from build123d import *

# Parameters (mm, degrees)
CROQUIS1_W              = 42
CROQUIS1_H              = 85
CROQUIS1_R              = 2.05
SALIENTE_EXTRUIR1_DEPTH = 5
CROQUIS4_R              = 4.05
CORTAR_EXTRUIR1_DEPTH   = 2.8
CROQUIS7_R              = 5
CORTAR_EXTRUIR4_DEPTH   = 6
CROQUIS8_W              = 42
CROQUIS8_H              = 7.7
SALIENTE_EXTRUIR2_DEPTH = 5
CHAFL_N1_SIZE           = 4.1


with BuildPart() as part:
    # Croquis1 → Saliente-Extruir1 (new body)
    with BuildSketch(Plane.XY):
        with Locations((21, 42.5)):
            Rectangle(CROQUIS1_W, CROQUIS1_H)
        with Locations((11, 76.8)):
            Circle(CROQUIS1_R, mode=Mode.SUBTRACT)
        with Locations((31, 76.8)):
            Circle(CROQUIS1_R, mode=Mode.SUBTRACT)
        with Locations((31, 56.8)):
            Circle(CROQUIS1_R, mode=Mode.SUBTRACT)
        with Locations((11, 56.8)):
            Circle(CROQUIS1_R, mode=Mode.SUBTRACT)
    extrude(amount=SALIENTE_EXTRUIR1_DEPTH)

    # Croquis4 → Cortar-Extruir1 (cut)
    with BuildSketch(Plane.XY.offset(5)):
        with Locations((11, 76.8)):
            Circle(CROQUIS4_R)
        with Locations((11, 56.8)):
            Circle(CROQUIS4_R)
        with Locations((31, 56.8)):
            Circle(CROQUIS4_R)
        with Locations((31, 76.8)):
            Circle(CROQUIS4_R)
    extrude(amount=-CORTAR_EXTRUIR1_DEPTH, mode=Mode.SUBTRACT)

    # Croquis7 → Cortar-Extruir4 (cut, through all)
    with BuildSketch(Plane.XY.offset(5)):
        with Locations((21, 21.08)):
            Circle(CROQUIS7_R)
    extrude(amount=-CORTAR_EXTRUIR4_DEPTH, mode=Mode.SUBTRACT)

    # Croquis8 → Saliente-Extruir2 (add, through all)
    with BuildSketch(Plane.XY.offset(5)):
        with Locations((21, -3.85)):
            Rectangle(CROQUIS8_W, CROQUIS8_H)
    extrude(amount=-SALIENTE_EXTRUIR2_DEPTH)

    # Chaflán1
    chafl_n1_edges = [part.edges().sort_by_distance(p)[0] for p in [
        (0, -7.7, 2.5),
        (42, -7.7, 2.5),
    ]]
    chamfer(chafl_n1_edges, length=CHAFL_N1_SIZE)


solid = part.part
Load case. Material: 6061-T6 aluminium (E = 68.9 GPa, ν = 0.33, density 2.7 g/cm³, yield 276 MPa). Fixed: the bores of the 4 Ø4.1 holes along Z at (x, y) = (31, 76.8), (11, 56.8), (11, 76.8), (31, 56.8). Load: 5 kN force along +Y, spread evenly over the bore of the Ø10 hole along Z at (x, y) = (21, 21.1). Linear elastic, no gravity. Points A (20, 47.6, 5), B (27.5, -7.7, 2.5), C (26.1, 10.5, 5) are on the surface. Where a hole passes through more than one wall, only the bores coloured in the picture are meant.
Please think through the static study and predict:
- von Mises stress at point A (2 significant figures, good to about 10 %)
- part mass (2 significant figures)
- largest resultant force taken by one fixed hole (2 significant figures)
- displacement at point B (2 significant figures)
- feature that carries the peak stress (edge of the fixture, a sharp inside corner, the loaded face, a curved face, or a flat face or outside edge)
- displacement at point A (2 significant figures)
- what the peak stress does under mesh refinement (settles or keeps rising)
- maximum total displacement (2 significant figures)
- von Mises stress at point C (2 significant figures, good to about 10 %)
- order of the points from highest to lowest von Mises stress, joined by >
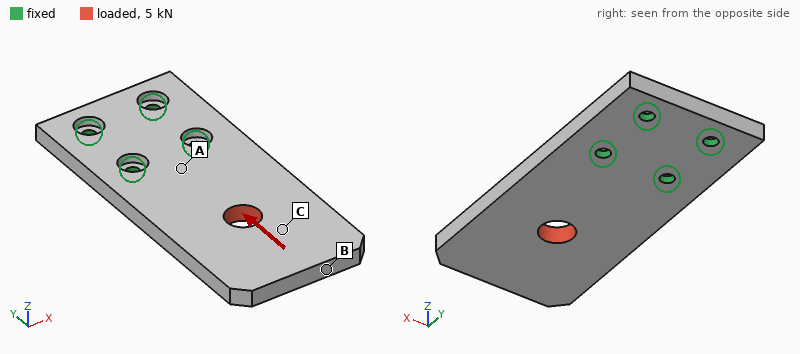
30 MPa
49 g
1.8 kN
89 µm
edge of the fixture
16 µm
keeps rising
90 µm
17 MPa
A > C > B
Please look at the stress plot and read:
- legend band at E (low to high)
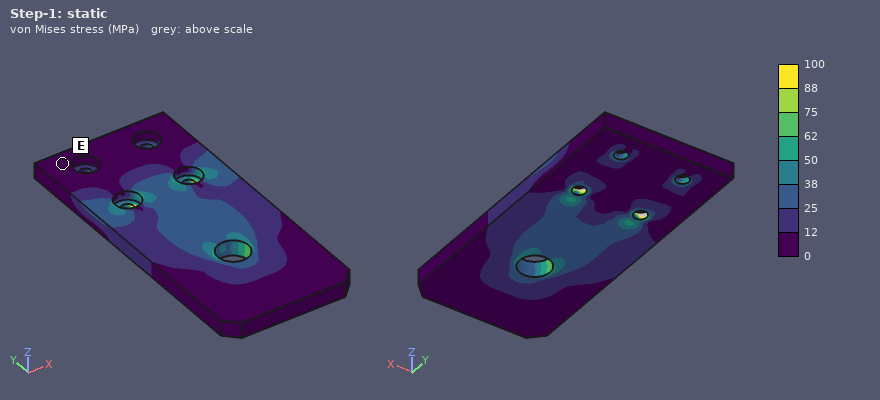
0 to 12 MPa
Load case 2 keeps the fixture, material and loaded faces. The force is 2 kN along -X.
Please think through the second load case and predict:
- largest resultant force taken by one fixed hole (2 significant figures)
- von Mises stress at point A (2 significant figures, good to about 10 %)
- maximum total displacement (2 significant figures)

2.3 kN
23 MPa
80 µm
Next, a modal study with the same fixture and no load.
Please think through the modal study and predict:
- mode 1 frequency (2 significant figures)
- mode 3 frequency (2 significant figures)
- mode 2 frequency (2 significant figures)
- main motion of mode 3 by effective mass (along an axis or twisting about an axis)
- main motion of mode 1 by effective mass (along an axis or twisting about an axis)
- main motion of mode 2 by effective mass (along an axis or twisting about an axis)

880 Hz
5200 Hz
3000 Hz
along X
along Z
twisting about Y
